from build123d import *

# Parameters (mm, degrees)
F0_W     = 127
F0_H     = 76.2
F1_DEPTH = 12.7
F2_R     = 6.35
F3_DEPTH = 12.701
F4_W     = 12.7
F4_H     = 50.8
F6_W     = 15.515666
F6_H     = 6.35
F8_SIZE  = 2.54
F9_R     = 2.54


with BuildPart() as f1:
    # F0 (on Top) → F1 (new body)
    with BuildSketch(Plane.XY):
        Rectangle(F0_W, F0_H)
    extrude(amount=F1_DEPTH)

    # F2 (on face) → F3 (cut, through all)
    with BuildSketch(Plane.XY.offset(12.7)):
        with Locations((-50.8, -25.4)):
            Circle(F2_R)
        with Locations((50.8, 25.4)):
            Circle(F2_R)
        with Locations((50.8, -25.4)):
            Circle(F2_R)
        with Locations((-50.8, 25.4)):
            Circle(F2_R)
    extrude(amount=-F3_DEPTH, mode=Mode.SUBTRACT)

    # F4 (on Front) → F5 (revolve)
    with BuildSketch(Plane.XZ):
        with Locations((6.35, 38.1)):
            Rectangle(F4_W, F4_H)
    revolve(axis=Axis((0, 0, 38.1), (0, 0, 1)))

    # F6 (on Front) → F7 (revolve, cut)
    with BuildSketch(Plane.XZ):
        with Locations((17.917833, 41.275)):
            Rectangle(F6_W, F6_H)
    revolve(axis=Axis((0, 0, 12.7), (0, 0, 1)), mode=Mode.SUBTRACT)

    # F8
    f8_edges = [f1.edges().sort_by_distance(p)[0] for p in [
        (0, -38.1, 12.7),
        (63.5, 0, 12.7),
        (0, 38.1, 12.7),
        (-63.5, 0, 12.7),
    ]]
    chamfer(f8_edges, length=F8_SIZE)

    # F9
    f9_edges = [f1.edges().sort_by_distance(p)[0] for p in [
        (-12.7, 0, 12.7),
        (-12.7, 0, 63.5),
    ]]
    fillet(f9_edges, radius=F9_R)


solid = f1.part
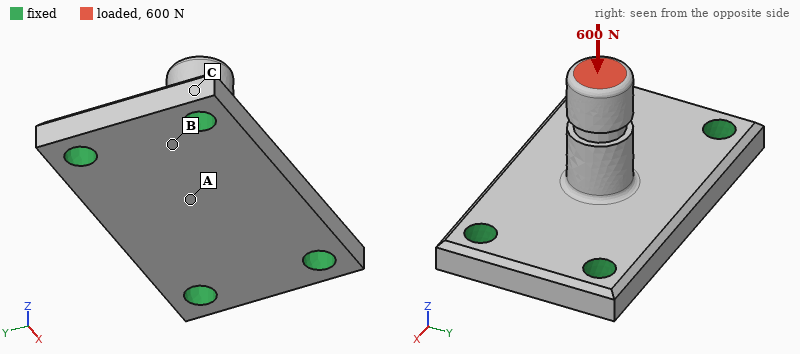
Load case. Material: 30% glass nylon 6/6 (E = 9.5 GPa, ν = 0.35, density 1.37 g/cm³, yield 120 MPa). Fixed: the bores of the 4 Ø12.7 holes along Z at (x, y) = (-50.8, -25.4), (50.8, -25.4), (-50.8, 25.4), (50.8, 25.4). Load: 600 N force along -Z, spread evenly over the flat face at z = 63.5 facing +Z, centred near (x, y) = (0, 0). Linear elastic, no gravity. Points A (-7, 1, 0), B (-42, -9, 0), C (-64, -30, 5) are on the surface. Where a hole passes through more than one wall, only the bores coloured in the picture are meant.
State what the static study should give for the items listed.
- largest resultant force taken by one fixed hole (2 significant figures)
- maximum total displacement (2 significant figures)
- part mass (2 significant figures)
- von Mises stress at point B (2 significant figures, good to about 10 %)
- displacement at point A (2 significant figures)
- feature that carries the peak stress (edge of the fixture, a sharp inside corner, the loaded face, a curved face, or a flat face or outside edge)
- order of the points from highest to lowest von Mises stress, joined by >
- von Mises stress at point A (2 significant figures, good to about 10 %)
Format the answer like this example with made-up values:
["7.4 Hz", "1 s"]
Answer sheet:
["150 N", "32 µm", "190 g", "1.3 MPa", "24 µm", "a curved face", "A > B > C", "2.5 MPa"]
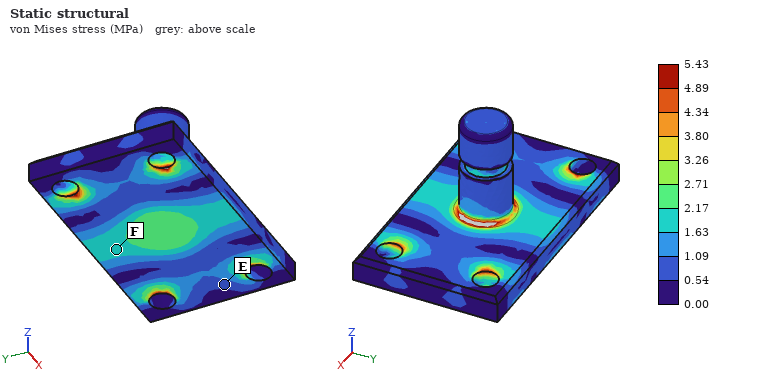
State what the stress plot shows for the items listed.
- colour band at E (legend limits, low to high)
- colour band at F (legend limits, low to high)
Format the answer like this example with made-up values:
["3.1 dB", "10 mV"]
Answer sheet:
["0.54 to 1.09 MPa", "1.63 to 2.17 MPa"]
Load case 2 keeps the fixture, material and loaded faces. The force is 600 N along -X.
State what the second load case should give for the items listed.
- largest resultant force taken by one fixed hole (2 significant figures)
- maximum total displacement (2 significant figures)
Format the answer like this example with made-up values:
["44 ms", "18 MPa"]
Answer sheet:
["290 N", "0.29 mm"]
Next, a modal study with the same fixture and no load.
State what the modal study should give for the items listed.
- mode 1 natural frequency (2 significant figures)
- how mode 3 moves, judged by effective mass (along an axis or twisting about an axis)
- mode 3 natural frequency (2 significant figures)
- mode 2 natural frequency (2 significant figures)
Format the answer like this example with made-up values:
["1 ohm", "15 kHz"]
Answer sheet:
["2000 Hz", "along Z", "2700 Hz", "2300 Hz"]
